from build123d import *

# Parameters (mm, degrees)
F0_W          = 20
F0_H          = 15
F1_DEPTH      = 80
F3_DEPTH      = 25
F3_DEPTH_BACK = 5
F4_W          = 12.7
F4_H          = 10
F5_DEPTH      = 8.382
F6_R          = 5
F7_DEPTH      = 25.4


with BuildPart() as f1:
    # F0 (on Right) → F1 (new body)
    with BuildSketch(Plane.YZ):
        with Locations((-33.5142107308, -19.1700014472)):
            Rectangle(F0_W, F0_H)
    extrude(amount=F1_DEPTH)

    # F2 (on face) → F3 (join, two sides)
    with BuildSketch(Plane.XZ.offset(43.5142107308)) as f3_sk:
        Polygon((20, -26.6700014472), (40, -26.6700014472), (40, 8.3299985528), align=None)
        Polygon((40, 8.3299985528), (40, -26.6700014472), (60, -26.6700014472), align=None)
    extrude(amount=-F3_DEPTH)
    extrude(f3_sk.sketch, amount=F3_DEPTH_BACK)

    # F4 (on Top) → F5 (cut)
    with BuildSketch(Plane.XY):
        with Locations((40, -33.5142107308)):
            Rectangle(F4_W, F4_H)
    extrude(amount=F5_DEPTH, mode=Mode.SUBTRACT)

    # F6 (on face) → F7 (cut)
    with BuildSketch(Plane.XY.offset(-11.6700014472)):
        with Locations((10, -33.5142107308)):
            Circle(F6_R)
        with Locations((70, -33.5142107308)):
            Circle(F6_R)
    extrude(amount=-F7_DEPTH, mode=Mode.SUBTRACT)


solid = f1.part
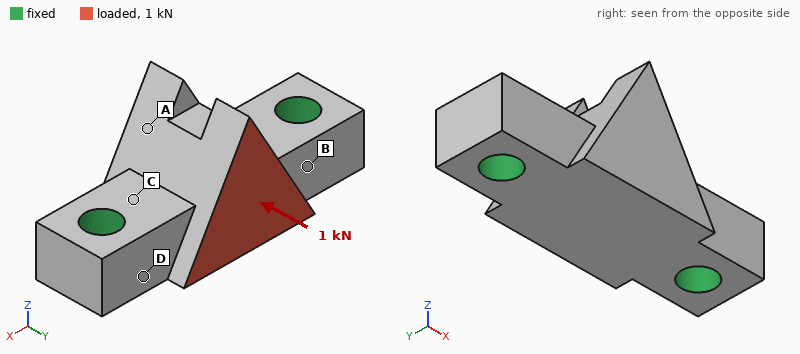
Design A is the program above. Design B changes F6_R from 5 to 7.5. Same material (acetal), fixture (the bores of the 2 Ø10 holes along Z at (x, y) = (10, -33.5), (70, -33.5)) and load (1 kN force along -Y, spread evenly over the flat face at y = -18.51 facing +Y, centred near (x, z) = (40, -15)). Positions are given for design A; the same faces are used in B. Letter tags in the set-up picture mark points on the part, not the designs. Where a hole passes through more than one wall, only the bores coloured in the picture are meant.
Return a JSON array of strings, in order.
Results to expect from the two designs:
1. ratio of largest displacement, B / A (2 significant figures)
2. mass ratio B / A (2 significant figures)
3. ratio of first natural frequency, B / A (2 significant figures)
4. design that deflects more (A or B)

["0.83", "0.91", "1.1", "A"]
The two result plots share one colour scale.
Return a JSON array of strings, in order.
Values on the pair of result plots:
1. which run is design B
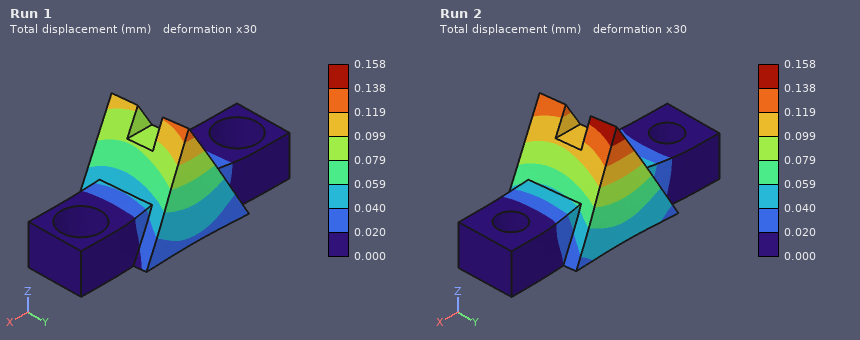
["Run 1"]
